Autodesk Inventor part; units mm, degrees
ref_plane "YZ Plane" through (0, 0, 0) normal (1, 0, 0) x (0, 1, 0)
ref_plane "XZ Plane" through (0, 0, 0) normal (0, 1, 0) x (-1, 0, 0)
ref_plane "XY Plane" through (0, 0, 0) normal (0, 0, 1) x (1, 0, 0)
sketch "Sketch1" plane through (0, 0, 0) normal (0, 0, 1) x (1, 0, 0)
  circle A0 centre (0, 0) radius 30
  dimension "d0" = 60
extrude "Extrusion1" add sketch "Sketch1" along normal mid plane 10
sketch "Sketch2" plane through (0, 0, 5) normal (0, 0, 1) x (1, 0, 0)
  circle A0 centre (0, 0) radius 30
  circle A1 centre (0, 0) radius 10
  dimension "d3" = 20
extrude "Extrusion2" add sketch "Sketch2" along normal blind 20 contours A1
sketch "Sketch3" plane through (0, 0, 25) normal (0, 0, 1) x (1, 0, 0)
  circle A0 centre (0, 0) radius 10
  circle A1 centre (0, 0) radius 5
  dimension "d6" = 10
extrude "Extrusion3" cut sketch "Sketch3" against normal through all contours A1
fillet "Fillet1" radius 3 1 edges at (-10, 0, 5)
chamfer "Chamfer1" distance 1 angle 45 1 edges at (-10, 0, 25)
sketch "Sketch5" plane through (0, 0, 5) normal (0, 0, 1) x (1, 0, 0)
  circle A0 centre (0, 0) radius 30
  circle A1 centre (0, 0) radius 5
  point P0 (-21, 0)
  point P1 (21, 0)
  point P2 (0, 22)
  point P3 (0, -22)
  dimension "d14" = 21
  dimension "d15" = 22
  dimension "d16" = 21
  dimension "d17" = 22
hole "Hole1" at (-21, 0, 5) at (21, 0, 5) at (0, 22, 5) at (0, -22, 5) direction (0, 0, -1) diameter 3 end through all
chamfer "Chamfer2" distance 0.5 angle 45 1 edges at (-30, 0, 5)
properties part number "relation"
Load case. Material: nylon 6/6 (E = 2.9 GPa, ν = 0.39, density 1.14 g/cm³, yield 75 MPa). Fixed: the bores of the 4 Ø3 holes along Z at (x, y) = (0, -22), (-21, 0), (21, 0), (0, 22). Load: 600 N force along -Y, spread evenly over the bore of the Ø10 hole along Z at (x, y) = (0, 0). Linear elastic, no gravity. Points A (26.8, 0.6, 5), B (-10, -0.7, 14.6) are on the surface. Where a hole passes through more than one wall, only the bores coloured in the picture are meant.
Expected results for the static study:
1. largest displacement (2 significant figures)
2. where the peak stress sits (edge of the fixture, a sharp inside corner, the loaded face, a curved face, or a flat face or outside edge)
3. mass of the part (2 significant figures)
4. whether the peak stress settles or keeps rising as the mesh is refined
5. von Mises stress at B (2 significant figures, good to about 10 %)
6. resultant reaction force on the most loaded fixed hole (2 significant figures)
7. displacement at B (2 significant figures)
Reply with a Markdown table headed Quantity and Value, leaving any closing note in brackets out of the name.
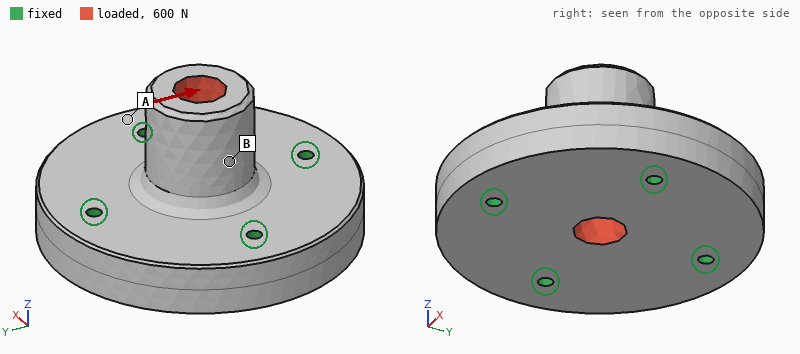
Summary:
| Quantity | Value |
|---|---|
| largest displacement | 79 µm |
| where the peak stress sits | edge of the fixture |
| mass of the part | 36 g |
| whether the peak stress settles or keeps rising as the mesh is refined | keeps rising |
| von Mises stress at B | 2.1 MPa |
| resultant reaction force on the most loaded fixed hole | 240 N |
| displacement at B | 41 µm |
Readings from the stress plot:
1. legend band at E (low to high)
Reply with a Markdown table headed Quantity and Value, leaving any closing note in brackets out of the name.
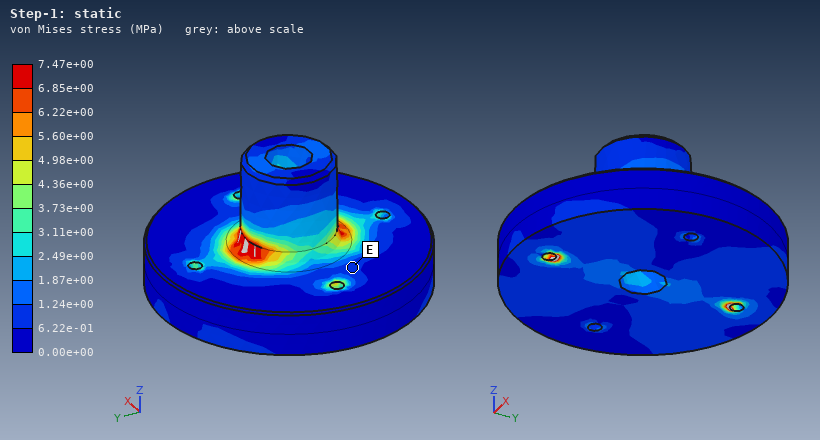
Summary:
| Quantity | Value |
|---|---|
| legend band at E | 6.22e-01 to 1.24e+00 MPa |
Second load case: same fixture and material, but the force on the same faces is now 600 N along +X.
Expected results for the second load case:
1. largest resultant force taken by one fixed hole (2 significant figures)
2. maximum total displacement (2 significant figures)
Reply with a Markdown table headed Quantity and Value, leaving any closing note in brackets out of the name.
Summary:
| Quantity | Value |
|---|---|
| largest resultant force taken by one fixed hole | 250 N |
| maximum total displacement | 78 µm |
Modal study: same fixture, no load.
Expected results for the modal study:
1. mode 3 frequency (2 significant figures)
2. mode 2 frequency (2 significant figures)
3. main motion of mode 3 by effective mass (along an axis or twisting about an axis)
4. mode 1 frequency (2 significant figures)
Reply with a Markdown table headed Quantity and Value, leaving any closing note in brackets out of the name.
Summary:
| Quantity | Value |
|---|---|
| mode 3 frequency | 6900 Hz |
| mode 2 frequency | 5600 Hz |
| main motion of mode 3 by effective mass | along Z |
| mode 1 frequency | 5500 Hz |
